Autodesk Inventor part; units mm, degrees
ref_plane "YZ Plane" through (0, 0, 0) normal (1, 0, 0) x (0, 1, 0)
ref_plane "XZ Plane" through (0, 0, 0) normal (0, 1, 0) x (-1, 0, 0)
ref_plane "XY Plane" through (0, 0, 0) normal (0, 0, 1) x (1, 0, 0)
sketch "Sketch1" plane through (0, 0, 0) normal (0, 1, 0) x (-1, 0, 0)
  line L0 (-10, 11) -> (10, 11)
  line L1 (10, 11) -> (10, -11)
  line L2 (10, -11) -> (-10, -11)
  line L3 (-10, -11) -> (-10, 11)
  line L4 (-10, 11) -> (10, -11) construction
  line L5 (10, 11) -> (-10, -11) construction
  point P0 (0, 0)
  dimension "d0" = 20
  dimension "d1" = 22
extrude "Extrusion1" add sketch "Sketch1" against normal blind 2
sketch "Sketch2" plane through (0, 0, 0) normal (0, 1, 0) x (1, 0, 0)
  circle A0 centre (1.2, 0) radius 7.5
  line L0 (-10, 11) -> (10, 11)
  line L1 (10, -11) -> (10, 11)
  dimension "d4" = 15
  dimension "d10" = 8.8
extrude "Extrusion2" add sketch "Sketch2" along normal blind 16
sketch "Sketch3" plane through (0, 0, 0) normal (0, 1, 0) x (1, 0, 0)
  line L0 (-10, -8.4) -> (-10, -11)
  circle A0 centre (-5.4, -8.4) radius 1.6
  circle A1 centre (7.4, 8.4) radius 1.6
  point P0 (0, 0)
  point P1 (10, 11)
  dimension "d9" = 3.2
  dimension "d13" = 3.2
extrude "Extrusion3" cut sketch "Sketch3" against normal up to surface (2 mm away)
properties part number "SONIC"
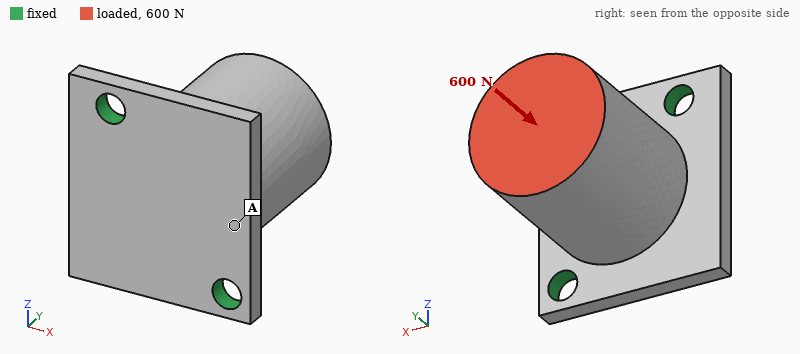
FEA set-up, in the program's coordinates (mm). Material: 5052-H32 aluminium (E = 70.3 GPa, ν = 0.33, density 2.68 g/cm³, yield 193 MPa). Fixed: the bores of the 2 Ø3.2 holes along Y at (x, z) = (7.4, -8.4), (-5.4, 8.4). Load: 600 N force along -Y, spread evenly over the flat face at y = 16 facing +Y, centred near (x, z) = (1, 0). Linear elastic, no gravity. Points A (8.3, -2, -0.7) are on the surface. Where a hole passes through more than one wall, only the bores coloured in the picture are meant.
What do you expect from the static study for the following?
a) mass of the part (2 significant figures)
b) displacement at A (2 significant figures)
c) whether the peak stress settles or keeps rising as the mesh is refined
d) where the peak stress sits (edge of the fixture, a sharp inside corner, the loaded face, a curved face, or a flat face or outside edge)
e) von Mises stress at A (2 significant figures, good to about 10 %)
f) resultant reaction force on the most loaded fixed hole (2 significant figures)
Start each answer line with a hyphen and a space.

- 9.8 g
- 6.5 µm
- keeps rising
- edge of the fixture
- 12 MPa
- 330 N
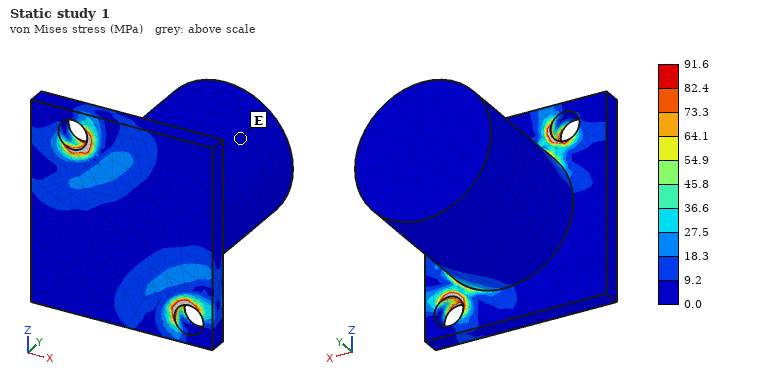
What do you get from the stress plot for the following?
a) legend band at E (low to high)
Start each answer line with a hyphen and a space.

- 0.0 to 9.2 MPa
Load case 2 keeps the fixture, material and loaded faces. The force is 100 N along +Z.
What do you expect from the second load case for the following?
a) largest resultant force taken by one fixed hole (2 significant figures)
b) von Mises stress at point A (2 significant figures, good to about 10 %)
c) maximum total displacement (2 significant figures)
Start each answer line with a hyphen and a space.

- 95 N
- 9.1 MPa
- 33 µm
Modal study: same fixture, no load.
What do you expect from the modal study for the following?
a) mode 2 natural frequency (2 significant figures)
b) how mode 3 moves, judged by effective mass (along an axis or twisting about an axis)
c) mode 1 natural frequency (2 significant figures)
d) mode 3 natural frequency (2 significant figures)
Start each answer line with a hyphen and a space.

- 14 kHz
- along Y
- 3900 Hz
- 17 kHz
